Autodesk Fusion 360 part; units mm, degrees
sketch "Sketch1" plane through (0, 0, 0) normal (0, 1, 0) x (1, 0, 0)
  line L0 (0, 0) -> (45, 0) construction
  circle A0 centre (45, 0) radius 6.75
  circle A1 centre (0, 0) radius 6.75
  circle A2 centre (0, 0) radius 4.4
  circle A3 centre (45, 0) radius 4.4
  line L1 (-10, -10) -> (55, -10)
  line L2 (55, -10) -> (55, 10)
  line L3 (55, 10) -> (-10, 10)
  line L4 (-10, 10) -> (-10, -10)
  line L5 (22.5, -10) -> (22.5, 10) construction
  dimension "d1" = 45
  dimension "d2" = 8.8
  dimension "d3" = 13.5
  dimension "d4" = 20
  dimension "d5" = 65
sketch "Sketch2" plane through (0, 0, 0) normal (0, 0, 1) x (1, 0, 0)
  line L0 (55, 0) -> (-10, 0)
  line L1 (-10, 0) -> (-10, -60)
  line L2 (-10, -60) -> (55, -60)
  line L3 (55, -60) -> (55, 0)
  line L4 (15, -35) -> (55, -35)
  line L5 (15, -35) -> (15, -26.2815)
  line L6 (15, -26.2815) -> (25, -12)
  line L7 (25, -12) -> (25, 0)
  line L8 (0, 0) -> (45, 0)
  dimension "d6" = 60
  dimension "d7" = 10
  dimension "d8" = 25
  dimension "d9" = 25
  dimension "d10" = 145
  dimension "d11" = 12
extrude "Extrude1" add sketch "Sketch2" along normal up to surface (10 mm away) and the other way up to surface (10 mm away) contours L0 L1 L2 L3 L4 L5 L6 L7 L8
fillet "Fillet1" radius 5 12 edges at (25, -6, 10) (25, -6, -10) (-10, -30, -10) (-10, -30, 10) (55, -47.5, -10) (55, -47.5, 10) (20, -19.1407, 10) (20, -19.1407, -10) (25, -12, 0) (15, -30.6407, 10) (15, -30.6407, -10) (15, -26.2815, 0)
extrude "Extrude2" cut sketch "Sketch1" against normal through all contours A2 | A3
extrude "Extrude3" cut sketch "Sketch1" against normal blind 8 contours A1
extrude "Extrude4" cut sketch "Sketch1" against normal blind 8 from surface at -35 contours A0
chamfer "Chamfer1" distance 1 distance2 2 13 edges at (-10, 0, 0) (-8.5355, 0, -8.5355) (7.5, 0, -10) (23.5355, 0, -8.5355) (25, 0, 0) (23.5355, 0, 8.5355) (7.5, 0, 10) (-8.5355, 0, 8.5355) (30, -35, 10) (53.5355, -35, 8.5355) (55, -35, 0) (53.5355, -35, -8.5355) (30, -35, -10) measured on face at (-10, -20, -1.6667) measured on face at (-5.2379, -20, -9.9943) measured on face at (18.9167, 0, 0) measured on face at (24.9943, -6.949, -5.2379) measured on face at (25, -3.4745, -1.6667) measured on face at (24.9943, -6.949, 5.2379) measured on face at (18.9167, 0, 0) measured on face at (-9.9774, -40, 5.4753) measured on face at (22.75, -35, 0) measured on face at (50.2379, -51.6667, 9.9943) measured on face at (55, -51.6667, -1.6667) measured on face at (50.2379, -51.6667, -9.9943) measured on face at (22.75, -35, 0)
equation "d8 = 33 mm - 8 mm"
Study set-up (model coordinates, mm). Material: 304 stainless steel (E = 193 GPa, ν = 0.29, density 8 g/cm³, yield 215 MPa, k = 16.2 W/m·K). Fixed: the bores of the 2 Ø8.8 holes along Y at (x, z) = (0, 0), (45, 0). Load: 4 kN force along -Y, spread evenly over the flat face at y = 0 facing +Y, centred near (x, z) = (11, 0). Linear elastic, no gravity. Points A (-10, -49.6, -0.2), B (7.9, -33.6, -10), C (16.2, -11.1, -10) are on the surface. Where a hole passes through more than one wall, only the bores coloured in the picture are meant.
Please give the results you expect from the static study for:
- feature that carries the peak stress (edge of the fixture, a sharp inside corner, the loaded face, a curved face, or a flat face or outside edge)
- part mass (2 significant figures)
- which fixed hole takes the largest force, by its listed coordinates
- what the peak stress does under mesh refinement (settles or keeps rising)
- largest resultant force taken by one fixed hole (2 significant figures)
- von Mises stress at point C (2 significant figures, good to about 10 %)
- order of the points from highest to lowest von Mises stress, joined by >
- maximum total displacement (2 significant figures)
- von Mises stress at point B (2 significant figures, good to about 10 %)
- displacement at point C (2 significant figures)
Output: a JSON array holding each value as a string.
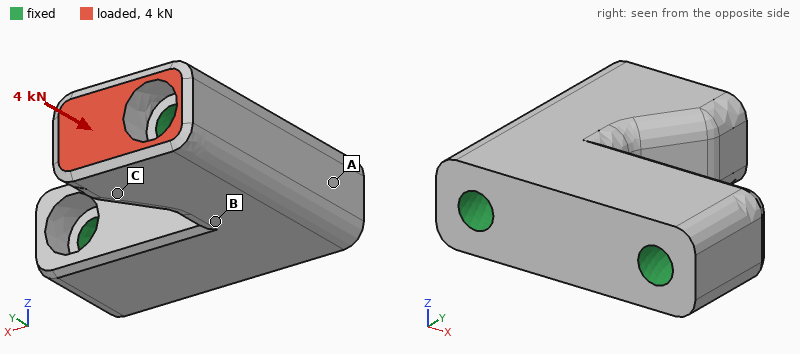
["edge of the fixture", "370 g", "(0, 0)", "keeps rising", "3.9 kN", "9.5 MPa", "C > B > A", "3.0 µm", "5.0 MPa", "1.6 µm"]
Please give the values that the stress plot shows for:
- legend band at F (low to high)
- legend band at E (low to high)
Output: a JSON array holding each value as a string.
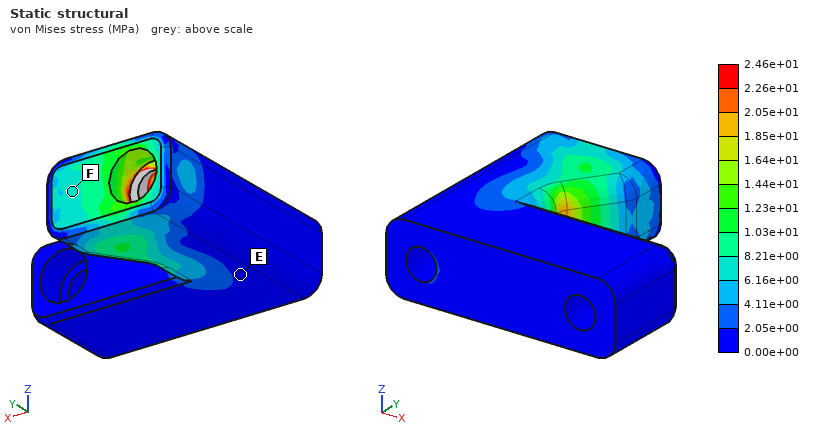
["6.16e+00 to 8.21e+00 MPa", "0.00e+00 to 2.05e+00 MPa"]
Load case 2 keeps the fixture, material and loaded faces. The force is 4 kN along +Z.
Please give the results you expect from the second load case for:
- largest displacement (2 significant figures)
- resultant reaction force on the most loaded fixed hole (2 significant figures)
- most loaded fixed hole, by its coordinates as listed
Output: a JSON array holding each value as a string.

["9.8 µm", "4.0 kN", "(0, 0)"]
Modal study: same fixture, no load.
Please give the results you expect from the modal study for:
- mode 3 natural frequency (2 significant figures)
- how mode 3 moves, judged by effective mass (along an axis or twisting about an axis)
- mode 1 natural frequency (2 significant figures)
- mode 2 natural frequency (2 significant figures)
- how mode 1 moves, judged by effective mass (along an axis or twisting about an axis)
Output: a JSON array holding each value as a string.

["26 kHz", "along Z", "18 kHz", "24 kHz", "along Z"]
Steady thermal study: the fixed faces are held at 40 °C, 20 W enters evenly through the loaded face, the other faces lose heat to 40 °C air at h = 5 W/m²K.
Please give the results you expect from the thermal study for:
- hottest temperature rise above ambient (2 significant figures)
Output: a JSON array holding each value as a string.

["57 K"]
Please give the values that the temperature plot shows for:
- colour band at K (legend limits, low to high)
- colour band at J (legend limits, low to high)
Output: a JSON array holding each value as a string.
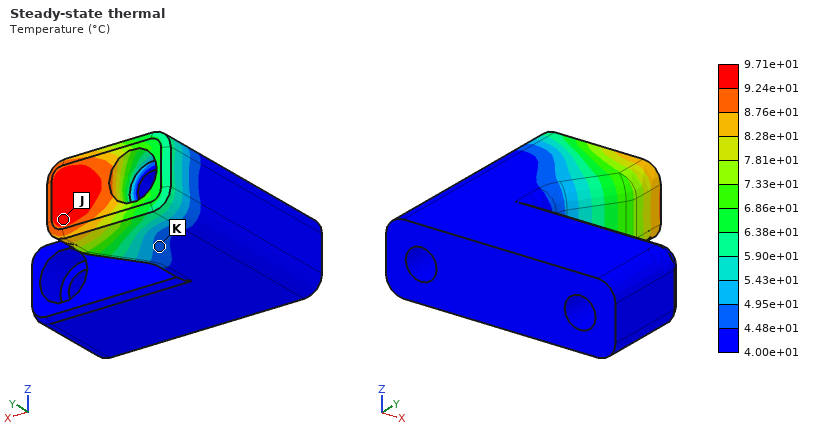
["4.48e+01 to 4.95e+01 °C", "9.24e+01 to 9.71e+01 °C"]
